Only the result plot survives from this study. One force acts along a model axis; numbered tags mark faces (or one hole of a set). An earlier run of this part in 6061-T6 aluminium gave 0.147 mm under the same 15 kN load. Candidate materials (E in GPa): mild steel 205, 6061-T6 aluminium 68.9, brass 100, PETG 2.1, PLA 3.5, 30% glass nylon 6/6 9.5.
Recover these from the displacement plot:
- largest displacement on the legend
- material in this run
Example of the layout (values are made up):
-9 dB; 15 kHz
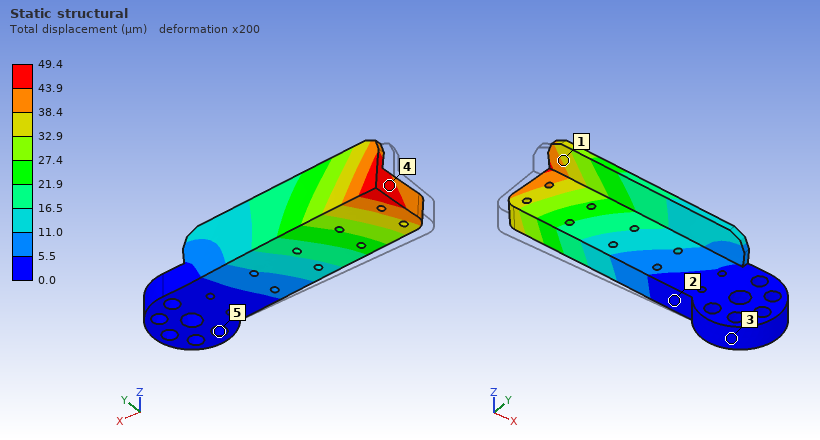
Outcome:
49.4 µm; mild steel
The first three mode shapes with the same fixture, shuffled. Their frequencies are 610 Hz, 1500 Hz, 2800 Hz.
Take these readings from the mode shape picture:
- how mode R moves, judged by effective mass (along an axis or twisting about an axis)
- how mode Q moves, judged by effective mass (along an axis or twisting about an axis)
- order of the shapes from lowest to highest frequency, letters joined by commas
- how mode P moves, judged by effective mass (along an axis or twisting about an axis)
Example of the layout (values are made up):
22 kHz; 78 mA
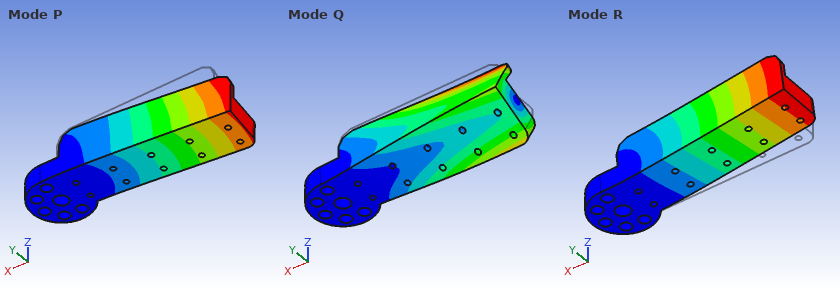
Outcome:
along Z; twisting about X; R, P, Q; along Y
